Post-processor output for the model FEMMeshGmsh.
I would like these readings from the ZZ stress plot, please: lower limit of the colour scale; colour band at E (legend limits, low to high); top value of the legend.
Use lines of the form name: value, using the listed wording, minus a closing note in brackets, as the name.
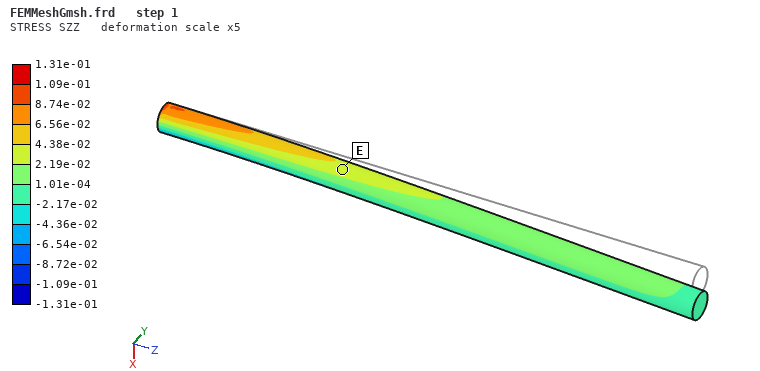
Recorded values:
lower limit of the colour scale: -1.31e-01
colour band at E: 2.19e-02 to 4.38e-02
top value of the legend: 1.31e-01
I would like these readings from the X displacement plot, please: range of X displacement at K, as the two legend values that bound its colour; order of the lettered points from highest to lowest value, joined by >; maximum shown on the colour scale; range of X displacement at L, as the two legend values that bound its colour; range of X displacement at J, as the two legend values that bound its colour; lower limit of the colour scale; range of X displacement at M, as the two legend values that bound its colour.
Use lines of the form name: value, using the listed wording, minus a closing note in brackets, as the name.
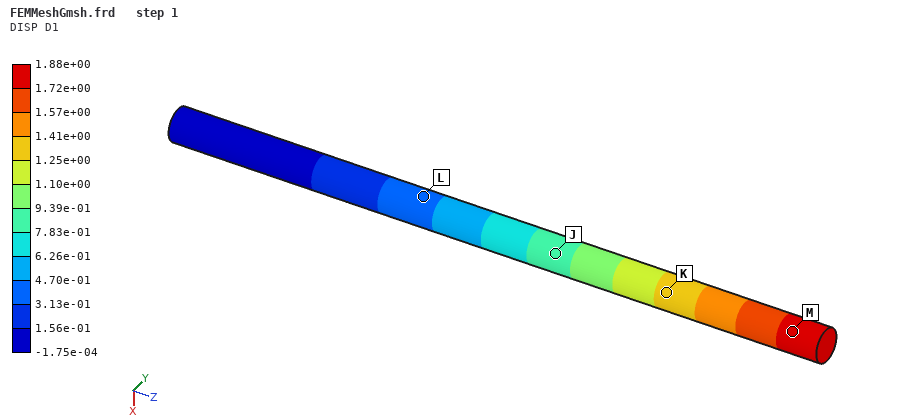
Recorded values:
range of X displacement at K, as the two legend values that bound its colour: 1.25e+00 to 1.41e+00
order of the lettered points from highest to lowest value, joined by >: M > K > J > L
maximum shown on the colour scale: 1.88e+00
range of X displacement at L, as the two legend values that bound its colour: 3.13e-01 to 4.70e-01
range of X displacement at J, as the two legend values that bound its colour: 7.83e-01 to 9.39e-01
lower limit of the colour scale: -1.75e-04
range of X displacement at M, as the two legend values that bound its colour: 1.72e+00 to 1.88e+00
